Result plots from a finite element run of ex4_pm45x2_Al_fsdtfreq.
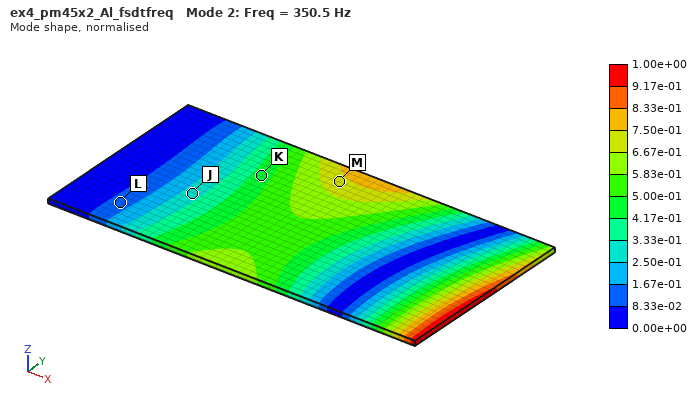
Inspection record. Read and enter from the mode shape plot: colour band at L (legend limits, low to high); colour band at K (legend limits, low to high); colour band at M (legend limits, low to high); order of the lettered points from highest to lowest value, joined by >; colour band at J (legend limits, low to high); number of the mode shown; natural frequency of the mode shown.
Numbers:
8.33e-02 to 1.67e-01
4.17e-01 to 5.00e-01
6.67e-01 to 7.50e-01
M > K > J > L
2.50e-01 to 3.33e-01
2
350.5 Hz
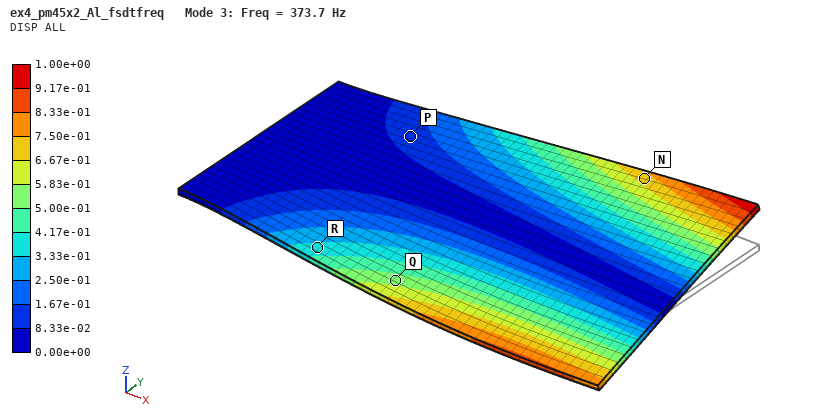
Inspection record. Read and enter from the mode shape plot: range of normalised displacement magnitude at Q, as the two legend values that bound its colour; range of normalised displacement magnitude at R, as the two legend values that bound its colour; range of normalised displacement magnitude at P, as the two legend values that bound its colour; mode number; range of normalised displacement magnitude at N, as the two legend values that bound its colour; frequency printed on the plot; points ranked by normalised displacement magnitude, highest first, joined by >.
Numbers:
5.00e-01 to 5.83e-01
3.33e-01 to 4.17e-01
8.33e-02 to 1.67e-01
3
6.67e-01 to 7.50e-01
373.7 Hz
N > Q > R > P
